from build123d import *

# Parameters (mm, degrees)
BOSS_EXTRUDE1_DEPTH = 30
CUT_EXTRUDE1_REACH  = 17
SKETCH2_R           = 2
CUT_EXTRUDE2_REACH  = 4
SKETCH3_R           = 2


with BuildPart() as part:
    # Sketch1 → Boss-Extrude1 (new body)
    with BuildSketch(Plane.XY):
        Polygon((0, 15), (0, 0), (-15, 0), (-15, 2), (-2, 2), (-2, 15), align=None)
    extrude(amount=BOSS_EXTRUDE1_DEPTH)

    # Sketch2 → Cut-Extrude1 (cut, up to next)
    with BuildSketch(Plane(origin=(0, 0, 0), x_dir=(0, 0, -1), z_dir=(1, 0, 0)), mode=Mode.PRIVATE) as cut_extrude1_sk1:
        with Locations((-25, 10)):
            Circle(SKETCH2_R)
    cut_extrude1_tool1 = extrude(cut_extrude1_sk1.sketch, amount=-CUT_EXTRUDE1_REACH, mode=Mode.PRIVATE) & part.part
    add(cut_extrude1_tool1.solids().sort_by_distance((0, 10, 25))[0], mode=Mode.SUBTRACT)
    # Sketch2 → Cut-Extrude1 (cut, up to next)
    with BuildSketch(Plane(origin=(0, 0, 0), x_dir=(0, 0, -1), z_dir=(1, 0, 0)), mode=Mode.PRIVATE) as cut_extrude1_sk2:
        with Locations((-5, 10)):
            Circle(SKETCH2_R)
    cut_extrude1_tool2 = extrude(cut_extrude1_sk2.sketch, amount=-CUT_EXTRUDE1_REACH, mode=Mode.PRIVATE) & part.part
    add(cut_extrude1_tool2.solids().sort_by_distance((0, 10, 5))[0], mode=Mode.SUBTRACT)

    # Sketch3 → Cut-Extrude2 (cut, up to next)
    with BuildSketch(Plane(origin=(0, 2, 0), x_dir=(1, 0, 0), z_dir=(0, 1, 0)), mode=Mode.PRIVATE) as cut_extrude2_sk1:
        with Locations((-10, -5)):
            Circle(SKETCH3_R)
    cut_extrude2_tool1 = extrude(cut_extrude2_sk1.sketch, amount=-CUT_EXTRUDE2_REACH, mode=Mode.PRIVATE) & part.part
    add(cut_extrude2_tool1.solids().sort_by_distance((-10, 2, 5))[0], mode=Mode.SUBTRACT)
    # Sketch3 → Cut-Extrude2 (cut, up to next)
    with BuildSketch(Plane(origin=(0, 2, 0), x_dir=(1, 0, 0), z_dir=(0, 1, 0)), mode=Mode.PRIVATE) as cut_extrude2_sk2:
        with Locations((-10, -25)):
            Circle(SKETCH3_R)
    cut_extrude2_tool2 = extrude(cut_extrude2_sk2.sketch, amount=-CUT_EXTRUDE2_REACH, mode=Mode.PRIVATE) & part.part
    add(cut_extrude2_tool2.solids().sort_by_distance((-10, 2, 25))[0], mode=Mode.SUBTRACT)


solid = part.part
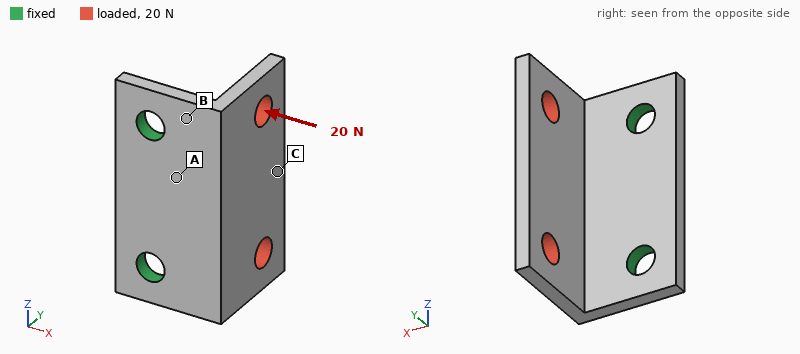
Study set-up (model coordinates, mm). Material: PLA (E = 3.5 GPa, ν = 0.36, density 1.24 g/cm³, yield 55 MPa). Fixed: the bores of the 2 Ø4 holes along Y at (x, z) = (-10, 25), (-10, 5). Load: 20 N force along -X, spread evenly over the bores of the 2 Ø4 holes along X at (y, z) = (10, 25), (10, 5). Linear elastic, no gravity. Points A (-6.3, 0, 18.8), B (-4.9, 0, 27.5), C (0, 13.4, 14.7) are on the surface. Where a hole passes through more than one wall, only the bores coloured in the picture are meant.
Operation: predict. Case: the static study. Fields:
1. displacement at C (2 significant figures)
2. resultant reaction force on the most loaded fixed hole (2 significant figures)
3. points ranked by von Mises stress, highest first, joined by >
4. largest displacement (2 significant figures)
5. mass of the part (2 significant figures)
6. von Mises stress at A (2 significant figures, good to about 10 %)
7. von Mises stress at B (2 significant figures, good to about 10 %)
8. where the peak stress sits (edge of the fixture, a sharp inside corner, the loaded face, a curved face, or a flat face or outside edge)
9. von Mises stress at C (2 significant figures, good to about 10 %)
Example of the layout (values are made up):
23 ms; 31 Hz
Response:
0.33 mm; 10 N; B > A > C; 0.40 mm; 2.0 g; 6.1 MPa; 8.7 MPa; a flat face or outside edge; 2.1 MPa
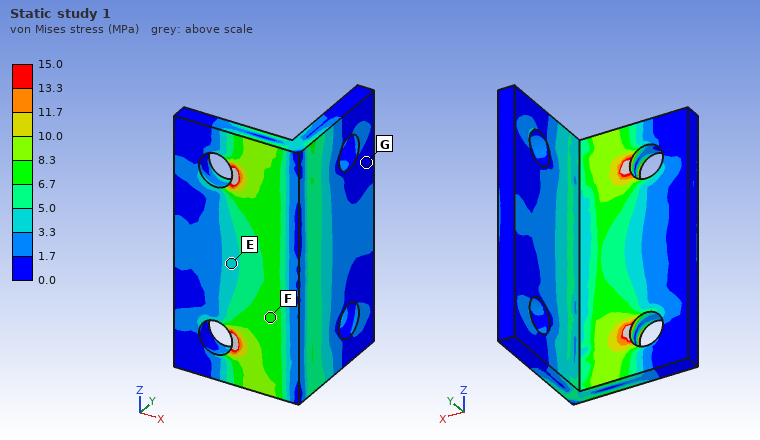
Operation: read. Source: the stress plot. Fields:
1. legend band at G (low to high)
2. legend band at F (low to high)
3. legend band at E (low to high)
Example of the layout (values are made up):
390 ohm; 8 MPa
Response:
0.0 to 1.7 MPa; 6.7 to 8.3 MPa; 3.3 to 5.0 MPa
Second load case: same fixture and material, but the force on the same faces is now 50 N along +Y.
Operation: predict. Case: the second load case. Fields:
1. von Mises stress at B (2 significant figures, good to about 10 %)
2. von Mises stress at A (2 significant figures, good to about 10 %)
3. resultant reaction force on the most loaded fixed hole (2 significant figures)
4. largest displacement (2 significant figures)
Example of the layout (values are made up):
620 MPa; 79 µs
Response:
11 MPa; 7.7 MPa; 25 N; 0.36 mm
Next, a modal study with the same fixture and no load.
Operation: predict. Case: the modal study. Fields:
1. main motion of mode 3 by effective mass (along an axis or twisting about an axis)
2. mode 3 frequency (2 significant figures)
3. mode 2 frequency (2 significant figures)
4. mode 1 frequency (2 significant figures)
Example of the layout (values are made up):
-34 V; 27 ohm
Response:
along Y; 4400 Hz; 2700 Hz; 1500 Hz
